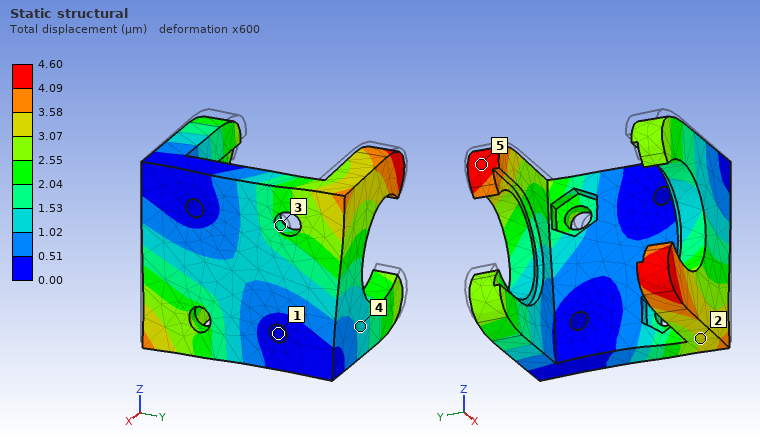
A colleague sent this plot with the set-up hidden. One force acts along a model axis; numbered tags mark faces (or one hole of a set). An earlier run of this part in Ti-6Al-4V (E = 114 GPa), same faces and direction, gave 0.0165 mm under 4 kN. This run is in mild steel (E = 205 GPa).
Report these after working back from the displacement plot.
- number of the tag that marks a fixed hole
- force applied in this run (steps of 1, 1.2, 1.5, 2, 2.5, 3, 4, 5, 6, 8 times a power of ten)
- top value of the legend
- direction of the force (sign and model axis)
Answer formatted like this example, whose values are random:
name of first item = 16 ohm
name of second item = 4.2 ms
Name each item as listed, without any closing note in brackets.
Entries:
number of the tag that marks a fixed hole = 1
force applied in this run = 2 kN
top value of the legend = 4.60 µm
direction of the force = +Y
